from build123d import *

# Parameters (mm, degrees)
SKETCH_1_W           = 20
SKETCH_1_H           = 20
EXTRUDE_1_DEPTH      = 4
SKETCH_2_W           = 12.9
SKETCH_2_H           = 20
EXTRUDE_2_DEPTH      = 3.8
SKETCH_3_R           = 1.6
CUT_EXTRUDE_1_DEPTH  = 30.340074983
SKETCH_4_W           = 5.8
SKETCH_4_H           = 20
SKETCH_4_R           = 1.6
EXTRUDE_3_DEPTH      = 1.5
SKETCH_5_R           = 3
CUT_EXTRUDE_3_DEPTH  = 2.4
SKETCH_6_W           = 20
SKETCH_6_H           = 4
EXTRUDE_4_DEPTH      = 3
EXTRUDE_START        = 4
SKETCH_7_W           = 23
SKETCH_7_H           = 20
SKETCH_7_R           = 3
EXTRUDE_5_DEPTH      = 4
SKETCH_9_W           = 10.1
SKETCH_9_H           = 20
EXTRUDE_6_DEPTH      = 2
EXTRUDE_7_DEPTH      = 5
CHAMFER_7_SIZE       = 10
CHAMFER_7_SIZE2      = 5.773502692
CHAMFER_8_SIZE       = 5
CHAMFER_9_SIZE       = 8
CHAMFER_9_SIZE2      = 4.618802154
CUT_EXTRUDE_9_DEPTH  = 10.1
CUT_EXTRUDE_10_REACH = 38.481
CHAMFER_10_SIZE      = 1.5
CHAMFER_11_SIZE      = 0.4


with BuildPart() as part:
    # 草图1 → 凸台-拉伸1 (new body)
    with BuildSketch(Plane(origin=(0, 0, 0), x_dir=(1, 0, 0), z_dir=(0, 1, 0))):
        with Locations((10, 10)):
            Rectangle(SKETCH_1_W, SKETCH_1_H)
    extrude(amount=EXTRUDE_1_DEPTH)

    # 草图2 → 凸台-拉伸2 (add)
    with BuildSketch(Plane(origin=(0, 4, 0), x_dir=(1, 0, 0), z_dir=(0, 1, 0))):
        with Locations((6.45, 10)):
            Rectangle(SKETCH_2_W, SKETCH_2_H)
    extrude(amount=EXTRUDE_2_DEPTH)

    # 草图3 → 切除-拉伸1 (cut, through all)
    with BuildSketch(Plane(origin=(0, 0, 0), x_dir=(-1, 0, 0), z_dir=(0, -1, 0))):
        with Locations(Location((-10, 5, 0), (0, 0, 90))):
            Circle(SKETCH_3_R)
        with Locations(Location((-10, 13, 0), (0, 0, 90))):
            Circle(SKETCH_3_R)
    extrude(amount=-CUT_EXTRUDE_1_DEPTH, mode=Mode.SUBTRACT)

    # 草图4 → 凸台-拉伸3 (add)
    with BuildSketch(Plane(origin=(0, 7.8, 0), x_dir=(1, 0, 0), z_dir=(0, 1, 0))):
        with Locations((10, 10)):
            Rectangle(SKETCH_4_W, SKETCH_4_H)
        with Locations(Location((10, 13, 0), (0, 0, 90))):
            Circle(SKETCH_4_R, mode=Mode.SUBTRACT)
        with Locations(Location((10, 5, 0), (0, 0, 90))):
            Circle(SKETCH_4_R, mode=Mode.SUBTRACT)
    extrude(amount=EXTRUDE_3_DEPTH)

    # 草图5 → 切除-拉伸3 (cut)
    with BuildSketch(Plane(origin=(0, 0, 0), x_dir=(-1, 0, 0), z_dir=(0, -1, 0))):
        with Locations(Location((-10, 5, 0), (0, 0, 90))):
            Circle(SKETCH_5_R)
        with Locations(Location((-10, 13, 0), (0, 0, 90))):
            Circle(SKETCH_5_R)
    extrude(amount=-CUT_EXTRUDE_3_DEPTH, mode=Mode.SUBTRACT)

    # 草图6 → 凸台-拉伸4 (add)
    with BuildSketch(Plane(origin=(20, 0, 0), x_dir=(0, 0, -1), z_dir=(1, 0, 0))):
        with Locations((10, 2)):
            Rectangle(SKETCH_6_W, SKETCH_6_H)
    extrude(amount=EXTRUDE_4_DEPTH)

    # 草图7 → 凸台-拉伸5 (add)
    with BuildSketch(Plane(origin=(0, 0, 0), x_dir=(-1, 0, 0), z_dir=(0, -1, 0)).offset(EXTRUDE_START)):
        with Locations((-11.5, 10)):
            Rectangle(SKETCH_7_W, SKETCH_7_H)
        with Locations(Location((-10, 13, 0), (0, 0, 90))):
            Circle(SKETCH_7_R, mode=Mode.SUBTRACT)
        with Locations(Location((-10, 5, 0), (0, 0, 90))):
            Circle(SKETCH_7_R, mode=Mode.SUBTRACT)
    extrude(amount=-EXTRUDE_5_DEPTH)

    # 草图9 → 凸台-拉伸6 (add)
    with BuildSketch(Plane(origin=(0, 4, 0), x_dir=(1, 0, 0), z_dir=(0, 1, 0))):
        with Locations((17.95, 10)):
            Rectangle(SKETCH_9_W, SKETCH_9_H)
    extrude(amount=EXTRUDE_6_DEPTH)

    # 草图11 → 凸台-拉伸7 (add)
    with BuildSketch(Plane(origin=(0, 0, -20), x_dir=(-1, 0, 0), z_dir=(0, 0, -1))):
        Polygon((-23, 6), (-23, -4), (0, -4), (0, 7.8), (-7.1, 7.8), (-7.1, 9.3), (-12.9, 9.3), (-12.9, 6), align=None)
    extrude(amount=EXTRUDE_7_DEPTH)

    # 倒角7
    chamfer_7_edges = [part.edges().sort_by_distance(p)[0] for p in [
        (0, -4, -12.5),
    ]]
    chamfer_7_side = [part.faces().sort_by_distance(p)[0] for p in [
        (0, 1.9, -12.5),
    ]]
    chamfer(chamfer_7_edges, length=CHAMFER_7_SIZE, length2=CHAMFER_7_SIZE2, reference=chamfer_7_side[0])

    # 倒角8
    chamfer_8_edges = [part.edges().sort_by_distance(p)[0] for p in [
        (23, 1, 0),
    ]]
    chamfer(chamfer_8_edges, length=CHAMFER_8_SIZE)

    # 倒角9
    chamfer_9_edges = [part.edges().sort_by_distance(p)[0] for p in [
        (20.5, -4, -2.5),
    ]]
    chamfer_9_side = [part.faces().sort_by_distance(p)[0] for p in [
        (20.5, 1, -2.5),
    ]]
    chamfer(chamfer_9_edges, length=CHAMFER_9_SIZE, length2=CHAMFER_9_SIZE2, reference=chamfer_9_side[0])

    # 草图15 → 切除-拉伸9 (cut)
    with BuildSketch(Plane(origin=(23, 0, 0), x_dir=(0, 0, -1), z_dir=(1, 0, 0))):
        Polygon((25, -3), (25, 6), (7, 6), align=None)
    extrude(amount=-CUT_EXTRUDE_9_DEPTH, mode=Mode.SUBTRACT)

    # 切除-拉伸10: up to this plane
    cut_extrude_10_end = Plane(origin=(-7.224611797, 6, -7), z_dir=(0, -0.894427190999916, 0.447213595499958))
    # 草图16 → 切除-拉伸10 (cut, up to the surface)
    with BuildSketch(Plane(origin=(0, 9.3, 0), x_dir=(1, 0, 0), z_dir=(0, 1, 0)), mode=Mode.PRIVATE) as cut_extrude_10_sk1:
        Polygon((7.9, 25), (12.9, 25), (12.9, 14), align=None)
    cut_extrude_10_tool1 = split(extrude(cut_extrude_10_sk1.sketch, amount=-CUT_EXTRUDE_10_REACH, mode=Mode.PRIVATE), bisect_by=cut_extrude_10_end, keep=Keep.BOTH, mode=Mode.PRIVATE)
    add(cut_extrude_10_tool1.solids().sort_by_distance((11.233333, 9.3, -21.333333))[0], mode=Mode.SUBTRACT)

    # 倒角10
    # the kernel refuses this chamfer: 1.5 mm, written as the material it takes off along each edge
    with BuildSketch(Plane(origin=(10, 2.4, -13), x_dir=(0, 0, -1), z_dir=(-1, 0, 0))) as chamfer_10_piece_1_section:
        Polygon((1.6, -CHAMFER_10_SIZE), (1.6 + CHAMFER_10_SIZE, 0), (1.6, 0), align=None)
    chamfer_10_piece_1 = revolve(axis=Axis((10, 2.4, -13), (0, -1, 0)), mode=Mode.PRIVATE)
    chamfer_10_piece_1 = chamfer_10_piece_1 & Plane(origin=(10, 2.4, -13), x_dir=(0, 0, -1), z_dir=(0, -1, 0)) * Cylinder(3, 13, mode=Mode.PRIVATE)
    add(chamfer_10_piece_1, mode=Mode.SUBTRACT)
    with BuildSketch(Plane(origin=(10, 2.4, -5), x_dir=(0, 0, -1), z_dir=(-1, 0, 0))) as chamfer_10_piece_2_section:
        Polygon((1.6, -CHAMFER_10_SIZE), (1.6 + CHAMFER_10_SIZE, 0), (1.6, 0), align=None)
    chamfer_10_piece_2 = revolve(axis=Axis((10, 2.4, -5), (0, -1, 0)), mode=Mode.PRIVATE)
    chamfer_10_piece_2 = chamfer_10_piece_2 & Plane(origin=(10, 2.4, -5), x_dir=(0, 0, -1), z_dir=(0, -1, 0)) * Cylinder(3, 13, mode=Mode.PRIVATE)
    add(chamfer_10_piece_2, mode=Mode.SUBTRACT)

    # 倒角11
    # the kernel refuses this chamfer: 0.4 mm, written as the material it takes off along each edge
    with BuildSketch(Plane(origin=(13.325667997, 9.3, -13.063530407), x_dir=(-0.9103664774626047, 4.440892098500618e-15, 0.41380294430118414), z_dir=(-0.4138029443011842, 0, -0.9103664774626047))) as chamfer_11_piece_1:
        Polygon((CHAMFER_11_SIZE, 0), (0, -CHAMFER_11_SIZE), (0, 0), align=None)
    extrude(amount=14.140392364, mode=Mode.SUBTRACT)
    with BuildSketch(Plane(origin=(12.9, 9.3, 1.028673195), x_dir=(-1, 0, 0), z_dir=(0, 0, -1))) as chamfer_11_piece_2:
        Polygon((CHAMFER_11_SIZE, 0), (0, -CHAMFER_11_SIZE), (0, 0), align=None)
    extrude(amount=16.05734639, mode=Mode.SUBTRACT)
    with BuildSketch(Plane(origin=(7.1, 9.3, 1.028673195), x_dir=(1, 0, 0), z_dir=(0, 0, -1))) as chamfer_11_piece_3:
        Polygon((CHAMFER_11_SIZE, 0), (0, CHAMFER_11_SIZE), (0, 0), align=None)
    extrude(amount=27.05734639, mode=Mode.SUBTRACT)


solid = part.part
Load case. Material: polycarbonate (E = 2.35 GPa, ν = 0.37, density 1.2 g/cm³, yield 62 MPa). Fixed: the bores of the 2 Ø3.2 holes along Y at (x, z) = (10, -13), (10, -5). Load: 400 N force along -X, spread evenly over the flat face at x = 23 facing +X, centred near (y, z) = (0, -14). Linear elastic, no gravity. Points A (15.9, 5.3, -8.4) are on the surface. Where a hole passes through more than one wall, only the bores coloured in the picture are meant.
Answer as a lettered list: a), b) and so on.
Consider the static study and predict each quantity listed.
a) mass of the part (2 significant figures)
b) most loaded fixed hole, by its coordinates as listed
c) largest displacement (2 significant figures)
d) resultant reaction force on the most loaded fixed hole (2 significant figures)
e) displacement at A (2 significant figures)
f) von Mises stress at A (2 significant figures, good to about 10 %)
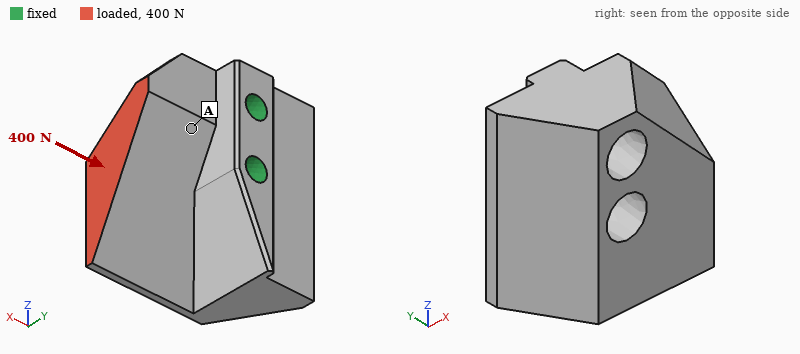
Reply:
a) 4.7 g
b) (10, -13)
c) 0.29 mm
d) 360 N
e) 0.067 mm
f) 6.3 MPa
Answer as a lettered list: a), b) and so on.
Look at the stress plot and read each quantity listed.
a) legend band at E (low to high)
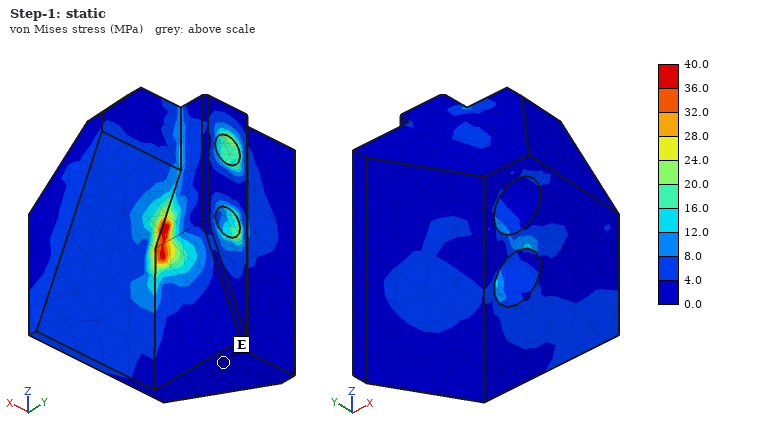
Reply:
a) 0.0 to 4.0 MPa
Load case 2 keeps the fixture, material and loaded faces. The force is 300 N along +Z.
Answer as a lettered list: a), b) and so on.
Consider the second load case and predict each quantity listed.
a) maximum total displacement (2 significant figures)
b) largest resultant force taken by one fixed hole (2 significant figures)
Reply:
a) 0.29 mm
b) 400 N
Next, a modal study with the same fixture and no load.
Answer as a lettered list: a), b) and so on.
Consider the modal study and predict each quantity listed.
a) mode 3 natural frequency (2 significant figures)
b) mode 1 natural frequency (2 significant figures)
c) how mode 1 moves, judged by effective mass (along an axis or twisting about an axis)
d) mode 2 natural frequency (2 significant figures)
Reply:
a) 7200 Hz
b) 4000 Hz
c) along X
d) 5500 Hz
